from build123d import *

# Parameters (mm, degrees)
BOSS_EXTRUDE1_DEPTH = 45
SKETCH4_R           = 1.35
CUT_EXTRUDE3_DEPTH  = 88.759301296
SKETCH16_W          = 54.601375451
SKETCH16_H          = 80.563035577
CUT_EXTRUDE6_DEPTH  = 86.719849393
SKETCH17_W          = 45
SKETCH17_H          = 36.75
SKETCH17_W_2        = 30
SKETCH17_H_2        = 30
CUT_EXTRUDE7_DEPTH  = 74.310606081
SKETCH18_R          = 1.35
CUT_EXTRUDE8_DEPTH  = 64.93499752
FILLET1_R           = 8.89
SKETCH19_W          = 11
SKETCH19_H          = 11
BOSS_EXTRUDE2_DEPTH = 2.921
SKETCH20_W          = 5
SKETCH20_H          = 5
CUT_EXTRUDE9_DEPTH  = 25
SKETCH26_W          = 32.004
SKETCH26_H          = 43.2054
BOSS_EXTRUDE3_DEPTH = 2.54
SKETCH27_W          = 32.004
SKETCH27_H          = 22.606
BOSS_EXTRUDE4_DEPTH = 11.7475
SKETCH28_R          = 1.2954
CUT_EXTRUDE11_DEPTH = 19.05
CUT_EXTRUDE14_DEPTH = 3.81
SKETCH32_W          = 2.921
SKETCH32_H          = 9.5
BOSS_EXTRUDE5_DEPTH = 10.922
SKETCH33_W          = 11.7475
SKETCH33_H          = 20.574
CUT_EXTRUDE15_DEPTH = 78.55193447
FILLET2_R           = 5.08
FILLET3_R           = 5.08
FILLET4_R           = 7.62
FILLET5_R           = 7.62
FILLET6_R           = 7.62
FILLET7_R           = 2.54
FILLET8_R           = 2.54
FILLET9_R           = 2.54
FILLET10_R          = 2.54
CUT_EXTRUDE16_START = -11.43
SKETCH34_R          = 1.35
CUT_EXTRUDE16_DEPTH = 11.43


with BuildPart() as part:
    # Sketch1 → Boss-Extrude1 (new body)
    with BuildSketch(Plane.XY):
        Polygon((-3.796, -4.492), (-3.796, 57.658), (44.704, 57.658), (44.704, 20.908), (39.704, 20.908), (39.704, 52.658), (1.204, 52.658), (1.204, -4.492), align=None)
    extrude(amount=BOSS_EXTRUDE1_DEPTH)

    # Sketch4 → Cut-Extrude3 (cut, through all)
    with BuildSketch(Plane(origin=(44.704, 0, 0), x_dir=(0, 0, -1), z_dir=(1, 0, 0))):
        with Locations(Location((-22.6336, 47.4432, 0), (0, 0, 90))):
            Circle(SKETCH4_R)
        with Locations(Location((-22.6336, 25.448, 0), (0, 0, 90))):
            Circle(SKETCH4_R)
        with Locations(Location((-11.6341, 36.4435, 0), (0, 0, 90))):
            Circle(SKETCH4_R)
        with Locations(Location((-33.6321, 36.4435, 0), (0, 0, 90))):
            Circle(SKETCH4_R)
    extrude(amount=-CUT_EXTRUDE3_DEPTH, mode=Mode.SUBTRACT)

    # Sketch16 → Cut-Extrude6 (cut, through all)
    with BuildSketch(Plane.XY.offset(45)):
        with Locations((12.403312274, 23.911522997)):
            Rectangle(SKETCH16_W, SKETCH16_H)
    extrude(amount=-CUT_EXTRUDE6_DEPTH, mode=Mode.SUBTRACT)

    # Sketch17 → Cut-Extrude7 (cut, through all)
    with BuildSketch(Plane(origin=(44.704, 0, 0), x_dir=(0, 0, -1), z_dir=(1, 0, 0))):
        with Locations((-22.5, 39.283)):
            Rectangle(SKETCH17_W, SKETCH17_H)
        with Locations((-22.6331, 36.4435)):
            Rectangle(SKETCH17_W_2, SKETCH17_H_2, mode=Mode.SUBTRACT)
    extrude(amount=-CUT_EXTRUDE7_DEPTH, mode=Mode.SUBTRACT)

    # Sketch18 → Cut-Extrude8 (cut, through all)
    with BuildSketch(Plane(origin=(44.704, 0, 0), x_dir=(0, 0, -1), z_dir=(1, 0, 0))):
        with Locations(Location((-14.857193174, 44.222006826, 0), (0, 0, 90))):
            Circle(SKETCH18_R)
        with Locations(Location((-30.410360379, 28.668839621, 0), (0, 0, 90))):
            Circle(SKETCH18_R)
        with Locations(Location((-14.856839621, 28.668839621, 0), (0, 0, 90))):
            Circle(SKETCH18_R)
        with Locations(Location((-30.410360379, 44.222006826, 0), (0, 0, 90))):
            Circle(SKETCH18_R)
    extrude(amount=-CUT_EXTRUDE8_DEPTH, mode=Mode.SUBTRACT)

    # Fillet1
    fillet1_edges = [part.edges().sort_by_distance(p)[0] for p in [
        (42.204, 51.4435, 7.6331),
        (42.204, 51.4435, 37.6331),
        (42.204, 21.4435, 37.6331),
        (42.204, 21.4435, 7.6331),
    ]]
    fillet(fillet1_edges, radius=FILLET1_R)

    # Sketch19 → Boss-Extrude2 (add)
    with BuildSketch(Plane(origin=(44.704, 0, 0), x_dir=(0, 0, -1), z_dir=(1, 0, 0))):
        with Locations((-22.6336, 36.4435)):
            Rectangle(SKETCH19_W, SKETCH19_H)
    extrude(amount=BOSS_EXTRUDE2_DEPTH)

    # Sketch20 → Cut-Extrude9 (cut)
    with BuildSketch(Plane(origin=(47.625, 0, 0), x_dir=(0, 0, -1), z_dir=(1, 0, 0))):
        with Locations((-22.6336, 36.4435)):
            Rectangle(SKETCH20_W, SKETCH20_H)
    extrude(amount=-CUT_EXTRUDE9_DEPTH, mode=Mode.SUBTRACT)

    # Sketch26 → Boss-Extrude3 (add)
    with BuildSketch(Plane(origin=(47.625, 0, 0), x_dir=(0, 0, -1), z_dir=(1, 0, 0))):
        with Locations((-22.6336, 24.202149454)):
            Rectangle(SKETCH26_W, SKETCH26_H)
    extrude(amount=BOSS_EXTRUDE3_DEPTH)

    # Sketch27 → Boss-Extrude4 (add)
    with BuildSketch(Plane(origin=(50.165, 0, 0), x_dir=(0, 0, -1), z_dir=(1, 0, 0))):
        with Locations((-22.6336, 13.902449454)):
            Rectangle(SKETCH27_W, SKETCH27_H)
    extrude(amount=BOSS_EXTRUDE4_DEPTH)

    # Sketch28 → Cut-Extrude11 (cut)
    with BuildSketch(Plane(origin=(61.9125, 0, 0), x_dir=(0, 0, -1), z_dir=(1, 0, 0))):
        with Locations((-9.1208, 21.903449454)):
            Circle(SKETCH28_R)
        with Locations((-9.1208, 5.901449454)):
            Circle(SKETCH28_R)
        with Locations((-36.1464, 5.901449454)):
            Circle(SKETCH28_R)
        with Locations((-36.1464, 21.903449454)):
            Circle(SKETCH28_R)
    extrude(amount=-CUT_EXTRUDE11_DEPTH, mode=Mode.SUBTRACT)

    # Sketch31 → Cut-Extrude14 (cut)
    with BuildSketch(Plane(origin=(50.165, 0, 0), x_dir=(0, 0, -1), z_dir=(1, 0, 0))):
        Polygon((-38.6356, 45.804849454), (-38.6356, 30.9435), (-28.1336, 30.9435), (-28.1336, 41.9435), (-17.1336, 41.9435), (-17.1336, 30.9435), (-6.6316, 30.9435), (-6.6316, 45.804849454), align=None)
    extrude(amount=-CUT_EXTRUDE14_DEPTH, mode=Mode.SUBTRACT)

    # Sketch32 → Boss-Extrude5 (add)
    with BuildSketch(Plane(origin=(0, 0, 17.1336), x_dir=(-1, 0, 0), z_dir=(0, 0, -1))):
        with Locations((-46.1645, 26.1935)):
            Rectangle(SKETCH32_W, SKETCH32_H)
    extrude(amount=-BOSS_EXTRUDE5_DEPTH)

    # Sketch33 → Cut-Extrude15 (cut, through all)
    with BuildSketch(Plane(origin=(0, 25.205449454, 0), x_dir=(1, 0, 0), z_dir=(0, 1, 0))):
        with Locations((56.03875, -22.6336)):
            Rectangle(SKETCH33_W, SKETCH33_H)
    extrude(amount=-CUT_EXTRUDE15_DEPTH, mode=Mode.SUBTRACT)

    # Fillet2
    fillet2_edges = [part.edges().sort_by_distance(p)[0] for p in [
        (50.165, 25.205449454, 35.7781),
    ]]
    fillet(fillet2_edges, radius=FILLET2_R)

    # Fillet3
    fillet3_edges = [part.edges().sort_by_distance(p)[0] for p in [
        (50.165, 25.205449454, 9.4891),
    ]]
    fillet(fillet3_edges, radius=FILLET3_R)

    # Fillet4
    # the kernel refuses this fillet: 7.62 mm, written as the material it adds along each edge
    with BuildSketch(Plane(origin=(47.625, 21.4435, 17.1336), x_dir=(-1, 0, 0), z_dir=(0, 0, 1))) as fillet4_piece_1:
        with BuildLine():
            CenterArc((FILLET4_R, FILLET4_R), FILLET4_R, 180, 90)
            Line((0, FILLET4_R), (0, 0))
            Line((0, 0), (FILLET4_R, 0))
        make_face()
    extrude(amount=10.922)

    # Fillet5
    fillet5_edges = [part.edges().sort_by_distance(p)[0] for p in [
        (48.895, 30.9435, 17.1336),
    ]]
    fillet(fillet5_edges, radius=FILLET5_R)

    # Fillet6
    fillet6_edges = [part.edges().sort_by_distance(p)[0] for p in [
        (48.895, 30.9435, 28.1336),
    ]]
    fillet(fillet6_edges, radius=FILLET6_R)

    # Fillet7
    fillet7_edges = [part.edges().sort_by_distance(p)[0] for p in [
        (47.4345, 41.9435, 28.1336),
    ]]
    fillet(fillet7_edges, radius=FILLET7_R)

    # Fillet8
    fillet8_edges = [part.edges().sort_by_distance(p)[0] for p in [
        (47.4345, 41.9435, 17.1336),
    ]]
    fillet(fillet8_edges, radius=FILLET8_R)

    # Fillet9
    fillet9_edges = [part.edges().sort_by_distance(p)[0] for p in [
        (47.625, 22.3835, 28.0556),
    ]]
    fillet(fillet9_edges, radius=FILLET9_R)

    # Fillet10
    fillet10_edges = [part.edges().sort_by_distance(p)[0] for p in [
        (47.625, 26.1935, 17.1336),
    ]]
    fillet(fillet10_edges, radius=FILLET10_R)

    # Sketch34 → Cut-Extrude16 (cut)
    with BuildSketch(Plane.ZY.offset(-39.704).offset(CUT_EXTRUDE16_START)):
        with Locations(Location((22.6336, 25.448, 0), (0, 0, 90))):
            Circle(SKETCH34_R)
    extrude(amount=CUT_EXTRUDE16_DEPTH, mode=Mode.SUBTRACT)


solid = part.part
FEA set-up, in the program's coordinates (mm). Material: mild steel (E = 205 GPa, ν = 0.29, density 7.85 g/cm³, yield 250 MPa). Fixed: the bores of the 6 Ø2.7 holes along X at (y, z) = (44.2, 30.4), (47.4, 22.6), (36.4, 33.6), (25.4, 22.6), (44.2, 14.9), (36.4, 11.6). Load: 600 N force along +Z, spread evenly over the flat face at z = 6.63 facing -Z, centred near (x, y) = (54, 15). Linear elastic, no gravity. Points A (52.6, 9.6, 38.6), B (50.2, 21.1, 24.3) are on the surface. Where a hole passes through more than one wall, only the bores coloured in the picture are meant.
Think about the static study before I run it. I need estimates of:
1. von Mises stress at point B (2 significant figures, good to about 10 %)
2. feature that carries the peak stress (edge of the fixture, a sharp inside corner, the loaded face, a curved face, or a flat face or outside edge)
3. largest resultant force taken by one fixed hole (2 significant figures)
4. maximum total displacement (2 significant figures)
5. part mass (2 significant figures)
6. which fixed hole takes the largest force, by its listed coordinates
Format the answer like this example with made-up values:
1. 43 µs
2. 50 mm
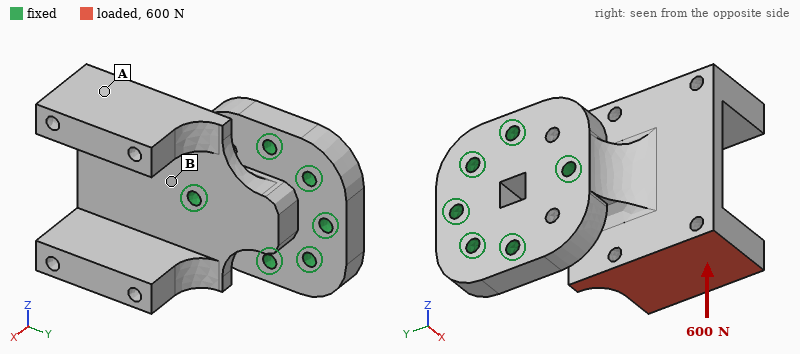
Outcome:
1. 28 MPa
2. a curved face
3. 800 N
4. 63 µm
5. 79 g
6. (25.4, 22.6)
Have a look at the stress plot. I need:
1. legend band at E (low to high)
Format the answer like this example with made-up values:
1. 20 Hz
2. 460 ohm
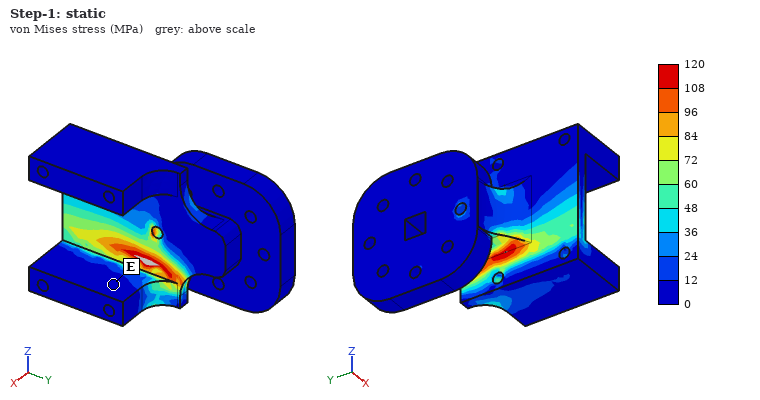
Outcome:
1. 0 to 12 MPa
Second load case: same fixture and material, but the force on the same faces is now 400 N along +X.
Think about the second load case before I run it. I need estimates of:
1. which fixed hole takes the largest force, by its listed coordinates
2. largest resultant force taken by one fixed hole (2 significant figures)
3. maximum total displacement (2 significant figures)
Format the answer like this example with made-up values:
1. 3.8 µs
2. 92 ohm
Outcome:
1. (25.4, 22.6)
2. 490 N
3. 76 µm
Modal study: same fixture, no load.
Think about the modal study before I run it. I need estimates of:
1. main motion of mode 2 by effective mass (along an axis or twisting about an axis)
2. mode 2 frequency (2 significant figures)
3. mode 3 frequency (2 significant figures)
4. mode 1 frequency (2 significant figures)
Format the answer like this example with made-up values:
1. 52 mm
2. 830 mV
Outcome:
1. along X
2. 4200 Hz
3. 6700 Hz
4. 3700 Hz
